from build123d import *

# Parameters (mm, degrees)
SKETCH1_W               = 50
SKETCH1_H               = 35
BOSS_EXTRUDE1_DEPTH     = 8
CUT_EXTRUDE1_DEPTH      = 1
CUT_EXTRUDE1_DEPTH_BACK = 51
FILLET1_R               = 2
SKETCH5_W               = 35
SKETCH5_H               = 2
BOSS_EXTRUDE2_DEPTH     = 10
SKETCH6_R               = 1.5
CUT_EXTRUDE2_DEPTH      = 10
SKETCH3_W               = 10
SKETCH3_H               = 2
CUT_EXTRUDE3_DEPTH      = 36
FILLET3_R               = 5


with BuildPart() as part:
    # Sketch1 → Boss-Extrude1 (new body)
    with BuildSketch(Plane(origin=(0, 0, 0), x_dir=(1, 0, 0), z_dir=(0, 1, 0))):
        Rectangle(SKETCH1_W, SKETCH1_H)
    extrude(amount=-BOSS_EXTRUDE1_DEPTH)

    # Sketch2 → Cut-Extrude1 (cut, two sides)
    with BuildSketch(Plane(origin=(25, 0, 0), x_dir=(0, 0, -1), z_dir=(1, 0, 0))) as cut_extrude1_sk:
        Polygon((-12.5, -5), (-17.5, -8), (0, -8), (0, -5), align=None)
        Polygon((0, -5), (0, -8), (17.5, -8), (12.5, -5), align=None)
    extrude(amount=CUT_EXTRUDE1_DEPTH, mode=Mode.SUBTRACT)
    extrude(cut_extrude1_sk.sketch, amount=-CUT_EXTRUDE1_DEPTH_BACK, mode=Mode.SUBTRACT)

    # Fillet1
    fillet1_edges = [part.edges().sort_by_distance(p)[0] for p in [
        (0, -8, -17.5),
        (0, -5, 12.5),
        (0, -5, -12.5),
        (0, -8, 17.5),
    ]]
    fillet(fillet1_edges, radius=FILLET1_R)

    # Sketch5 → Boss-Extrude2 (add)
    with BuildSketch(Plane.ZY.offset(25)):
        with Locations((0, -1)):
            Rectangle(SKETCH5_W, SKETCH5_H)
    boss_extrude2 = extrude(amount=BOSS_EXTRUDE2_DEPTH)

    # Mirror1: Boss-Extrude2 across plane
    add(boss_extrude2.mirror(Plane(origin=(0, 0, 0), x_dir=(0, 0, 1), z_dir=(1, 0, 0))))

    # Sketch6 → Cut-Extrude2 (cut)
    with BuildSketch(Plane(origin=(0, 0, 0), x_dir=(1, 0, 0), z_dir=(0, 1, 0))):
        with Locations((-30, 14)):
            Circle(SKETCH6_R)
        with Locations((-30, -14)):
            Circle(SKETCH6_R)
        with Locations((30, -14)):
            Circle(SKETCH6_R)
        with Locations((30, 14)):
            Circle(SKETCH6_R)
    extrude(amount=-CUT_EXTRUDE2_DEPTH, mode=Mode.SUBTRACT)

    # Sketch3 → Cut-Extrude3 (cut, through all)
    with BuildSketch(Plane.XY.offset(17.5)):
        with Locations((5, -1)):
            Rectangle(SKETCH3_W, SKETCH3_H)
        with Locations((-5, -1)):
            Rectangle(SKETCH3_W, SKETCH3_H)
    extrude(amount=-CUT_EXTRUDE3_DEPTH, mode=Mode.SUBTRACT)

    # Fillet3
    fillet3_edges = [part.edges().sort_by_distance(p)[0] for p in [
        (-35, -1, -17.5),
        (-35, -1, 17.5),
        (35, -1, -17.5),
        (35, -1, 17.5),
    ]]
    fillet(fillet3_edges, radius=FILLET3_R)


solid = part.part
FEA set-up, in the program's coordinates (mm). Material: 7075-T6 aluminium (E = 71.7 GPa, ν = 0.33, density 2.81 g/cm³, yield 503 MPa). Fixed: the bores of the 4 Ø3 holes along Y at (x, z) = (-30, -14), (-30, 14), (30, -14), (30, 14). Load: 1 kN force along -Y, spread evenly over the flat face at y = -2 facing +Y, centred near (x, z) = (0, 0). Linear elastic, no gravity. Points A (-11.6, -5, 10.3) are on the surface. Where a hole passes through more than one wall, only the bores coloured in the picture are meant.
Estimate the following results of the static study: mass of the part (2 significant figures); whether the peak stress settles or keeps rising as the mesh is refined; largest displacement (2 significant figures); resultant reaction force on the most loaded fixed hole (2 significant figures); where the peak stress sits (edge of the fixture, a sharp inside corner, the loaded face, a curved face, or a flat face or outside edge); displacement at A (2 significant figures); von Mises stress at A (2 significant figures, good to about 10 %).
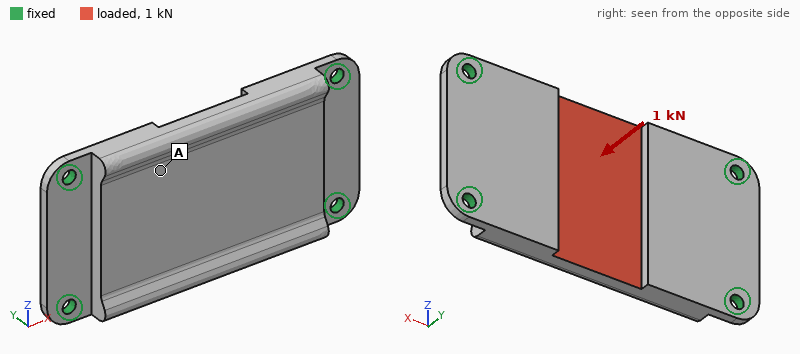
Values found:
26 g
keeps rising
0.11 mm
1.1 kN
edge of the fixture
0.075 mm
28 MPa
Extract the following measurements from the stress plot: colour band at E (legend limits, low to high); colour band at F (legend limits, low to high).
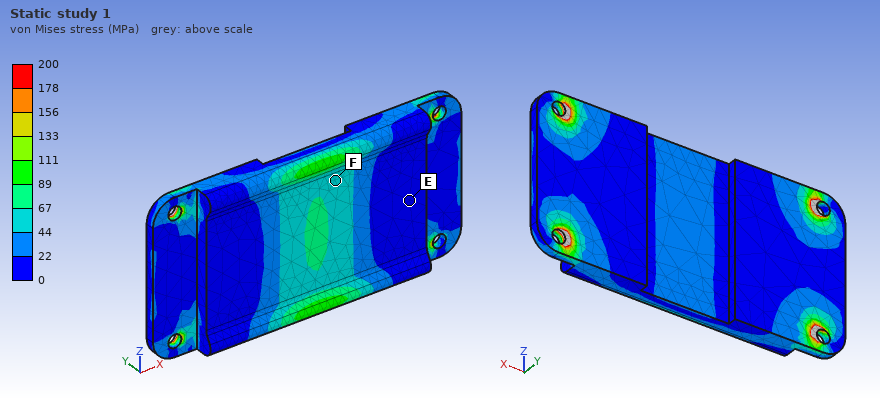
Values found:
0 to 22 MPa
44 to 67 MPa
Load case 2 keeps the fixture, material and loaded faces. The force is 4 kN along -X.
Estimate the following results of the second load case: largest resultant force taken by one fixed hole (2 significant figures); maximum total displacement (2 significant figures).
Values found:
1.0 kN
20 µm
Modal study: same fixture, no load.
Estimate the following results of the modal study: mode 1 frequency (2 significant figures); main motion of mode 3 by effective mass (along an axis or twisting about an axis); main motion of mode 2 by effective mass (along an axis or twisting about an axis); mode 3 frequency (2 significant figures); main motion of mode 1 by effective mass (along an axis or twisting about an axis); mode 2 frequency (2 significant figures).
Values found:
4800 Hz
twisting about Z
twisting about X
11 kHz
along Y
8100 Hz
